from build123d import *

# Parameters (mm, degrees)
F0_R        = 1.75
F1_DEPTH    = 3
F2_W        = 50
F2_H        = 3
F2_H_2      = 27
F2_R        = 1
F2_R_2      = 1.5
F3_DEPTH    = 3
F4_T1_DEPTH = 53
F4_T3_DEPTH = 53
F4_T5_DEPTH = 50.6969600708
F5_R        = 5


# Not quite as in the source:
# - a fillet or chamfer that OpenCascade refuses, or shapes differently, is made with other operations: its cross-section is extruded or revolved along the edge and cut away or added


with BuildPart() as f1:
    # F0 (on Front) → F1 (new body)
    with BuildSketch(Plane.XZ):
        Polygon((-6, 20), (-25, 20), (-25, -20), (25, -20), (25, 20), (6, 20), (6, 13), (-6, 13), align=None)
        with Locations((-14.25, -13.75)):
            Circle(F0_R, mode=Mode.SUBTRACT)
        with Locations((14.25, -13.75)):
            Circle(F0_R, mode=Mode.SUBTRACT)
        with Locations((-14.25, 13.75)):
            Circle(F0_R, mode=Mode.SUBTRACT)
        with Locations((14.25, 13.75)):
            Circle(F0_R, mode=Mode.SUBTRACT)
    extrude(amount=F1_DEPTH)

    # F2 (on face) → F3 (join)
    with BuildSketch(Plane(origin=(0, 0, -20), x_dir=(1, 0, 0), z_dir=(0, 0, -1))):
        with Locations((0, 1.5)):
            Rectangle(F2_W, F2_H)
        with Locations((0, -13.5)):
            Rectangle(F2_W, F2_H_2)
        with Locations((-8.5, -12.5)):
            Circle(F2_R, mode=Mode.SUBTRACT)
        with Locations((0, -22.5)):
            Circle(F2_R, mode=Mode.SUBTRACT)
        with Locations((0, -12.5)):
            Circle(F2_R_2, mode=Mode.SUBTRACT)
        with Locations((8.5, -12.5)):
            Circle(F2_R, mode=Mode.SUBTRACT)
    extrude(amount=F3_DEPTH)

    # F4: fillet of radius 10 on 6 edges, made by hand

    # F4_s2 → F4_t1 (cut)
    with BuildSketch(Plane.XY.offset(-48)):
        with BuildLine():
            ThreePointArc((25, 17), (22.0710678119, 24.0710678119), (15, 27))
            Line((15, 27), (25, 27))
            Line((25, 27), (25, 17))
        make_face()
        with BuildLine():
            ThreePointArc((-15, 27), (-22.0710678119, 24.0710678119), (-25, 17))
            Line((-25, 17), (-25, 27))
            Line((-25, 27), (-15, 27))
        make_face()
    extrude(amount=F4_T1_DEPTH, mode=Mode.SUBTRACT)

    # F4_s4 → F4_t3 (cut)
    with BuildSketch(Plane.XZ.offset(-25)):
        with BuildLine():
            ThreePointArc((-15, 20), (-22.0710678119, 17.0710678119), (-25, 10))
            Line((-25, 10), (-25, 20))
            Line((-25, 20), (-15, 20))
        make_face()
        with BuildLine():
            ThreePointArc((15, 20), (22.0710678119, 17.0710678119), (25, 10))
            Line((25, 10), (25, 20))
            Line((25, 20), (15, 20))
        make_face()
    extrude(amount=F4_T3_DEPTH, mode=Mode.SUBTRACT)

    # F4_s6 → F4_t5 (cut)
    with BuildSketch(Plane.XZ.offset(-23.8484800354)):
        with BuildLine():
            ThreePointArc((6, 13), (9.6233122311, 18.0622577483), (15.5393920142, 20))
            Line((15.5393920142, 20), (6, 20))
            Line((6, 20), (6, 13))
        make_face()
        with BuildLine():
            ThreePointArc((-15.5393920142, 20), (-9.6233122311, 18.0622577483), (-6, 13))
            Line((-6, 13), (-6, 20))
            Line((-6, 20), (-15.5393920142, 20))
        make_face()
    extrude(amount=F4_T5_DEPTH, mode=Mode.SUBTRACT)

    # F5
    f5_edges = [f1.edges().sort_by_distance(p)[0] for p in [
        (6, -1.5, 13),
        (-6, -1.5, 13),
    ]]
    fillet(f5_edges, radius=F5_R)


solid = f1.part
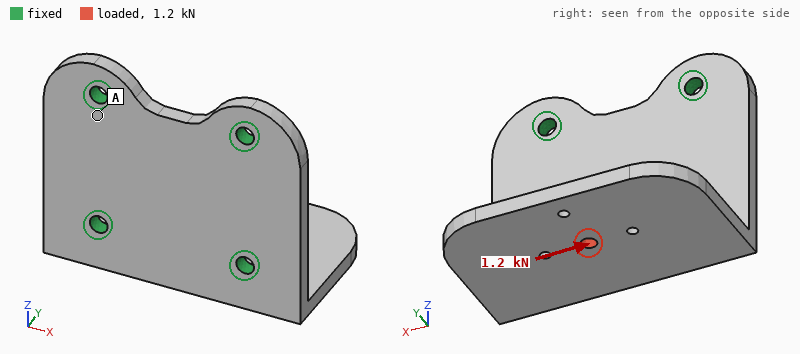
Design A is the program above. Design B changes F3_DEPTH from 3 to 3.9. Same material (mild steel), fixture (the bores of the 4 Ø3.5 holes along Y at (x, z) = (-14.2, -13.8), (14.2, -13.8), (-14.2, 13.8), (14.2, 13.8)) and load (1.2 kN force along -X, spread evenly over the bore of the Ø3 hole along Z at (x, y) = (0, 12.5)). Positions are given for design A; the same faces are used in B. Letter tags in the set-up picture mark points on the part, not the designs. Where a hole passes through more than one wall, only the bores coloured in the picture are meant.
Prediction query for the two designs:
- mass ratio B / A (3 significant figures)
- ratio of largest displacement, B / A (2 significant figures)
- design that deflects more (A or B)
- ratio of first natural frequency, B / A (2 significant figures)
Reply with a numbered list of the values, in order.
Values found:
1. 1.13
2. 0.85
3. A
4. 0.98
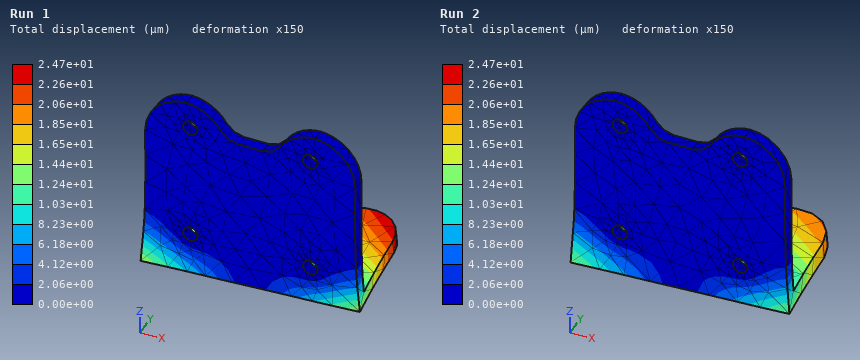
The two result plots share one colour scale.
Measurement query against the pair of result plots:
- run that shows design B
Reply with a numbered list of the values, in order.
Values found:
1. Run 2
